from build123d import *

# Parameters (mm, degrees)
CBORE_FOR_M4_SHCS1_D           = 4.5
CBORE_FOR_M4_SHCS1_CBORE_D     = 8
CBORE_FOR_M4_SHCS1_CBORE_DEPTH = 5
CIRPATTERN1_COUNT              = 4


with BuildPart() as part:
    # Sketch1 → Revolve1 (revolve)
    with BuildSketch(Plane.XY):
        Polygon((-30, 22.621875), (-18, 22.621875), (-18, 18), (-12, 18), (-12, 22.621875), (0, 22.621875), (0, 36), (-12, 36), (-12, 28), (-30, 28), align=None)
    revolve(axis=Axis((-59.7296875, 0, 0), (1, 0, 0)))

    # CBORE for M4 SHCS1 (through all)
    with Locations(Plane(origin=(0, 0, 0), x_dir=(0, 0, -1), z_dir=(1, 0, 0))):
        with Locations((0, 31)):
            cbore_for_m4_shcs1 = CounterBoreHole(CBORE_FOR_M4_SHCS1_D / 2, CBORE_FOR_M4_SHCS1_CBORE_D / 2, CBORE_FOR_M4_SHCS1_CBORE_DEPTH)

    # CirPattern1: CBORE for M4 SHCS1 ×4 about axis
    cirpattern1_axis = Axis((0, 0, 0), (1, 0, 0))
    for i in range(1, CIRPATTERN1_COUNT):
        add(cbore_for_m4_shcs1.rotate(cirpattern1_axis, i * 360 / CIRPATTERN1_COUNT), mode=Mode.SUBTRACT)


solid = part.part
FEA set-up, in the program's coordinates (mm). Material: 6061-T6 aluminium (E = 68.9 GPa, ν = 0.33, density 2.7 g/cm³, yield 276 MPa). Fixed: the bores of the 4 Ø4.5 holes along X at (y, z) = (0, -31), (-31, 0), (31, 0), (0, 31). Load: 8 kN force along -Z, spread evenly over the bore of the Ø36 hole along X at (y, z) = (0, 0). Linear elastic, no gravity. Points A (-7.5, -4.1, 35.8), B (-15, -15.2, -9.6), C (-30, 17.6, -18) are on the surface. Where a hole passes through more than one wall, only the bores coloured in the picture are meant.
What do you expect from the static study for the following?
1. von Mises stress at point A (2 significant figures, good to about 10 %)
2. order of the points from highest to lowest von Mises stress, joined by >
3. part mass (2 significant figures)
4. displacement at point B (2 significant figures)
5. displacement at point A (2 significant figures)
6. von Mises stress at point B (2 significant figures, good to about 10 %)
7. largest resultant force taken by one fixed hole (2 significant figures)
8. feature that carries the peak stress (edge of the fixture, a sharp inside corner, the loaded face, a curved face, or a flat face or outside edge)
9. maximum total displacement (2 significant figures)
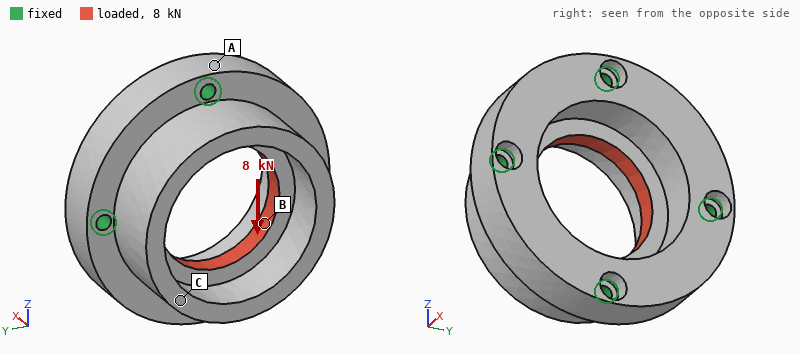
11 MPa
B > A > C
130 g
7.7 µm
1.3 µm
19 MPa
2.3 kN
edge of the fixture
8.2 µm
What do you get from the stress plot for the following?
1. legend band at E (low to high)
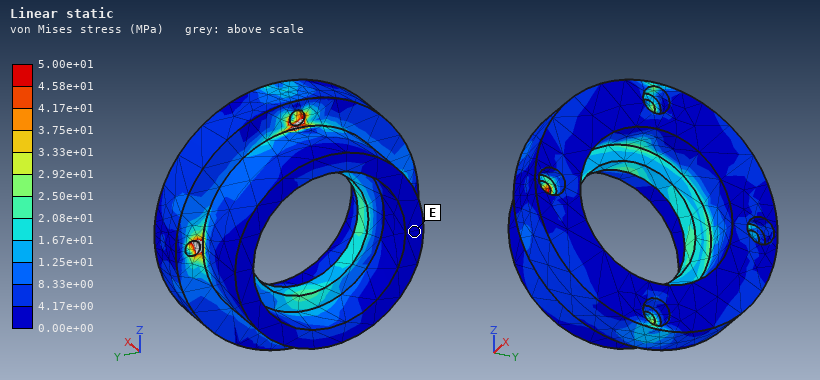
0.00e+00 to 4.17e+00 MPa
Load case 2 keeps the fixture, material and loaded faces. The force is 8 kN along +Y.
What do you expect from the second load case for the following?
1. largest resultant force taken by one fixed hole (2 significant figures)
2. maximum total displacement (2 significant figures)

2.3 kN
8.2 µm
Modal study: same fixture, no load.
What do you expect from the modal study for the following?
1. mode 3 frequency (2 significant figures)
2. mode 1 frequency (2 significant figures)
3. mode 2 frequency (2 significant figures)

15 kHz
11 kHz
15 kHz
